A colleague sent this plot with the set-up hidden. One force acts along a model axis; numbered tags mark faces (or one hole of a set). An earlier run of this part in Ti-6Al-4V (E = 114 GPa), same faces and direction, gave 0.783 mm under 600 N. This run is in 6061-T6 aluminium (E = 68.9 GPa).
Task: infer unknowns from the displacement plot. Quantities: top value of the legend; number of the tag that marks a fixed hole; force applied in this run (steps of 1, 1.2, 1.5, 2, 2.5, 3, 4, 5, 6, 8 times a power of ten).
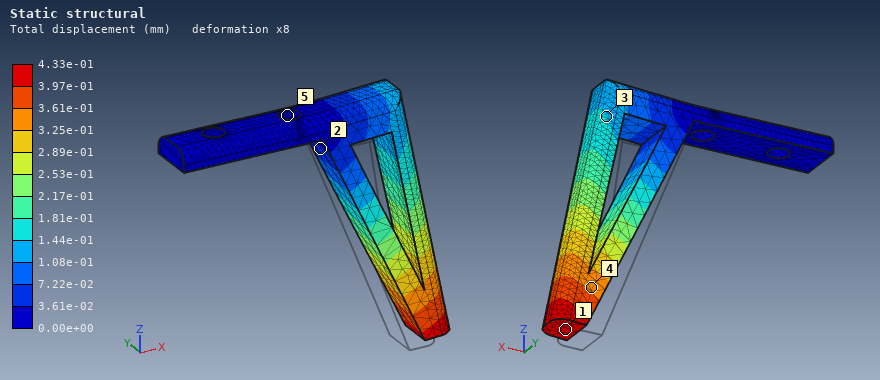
4.33e-01 mm
5
200 N
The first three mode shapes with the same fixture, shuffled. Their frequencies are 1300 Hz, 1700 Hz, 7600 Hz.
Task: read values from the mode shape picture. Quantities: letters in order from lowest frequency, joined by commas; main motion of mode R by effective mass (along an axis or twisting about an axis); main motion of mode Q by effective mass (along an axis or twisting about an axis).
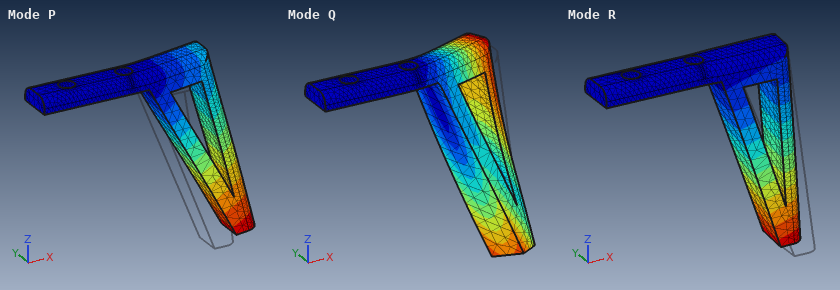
P, R, Q
along Y
along Y
